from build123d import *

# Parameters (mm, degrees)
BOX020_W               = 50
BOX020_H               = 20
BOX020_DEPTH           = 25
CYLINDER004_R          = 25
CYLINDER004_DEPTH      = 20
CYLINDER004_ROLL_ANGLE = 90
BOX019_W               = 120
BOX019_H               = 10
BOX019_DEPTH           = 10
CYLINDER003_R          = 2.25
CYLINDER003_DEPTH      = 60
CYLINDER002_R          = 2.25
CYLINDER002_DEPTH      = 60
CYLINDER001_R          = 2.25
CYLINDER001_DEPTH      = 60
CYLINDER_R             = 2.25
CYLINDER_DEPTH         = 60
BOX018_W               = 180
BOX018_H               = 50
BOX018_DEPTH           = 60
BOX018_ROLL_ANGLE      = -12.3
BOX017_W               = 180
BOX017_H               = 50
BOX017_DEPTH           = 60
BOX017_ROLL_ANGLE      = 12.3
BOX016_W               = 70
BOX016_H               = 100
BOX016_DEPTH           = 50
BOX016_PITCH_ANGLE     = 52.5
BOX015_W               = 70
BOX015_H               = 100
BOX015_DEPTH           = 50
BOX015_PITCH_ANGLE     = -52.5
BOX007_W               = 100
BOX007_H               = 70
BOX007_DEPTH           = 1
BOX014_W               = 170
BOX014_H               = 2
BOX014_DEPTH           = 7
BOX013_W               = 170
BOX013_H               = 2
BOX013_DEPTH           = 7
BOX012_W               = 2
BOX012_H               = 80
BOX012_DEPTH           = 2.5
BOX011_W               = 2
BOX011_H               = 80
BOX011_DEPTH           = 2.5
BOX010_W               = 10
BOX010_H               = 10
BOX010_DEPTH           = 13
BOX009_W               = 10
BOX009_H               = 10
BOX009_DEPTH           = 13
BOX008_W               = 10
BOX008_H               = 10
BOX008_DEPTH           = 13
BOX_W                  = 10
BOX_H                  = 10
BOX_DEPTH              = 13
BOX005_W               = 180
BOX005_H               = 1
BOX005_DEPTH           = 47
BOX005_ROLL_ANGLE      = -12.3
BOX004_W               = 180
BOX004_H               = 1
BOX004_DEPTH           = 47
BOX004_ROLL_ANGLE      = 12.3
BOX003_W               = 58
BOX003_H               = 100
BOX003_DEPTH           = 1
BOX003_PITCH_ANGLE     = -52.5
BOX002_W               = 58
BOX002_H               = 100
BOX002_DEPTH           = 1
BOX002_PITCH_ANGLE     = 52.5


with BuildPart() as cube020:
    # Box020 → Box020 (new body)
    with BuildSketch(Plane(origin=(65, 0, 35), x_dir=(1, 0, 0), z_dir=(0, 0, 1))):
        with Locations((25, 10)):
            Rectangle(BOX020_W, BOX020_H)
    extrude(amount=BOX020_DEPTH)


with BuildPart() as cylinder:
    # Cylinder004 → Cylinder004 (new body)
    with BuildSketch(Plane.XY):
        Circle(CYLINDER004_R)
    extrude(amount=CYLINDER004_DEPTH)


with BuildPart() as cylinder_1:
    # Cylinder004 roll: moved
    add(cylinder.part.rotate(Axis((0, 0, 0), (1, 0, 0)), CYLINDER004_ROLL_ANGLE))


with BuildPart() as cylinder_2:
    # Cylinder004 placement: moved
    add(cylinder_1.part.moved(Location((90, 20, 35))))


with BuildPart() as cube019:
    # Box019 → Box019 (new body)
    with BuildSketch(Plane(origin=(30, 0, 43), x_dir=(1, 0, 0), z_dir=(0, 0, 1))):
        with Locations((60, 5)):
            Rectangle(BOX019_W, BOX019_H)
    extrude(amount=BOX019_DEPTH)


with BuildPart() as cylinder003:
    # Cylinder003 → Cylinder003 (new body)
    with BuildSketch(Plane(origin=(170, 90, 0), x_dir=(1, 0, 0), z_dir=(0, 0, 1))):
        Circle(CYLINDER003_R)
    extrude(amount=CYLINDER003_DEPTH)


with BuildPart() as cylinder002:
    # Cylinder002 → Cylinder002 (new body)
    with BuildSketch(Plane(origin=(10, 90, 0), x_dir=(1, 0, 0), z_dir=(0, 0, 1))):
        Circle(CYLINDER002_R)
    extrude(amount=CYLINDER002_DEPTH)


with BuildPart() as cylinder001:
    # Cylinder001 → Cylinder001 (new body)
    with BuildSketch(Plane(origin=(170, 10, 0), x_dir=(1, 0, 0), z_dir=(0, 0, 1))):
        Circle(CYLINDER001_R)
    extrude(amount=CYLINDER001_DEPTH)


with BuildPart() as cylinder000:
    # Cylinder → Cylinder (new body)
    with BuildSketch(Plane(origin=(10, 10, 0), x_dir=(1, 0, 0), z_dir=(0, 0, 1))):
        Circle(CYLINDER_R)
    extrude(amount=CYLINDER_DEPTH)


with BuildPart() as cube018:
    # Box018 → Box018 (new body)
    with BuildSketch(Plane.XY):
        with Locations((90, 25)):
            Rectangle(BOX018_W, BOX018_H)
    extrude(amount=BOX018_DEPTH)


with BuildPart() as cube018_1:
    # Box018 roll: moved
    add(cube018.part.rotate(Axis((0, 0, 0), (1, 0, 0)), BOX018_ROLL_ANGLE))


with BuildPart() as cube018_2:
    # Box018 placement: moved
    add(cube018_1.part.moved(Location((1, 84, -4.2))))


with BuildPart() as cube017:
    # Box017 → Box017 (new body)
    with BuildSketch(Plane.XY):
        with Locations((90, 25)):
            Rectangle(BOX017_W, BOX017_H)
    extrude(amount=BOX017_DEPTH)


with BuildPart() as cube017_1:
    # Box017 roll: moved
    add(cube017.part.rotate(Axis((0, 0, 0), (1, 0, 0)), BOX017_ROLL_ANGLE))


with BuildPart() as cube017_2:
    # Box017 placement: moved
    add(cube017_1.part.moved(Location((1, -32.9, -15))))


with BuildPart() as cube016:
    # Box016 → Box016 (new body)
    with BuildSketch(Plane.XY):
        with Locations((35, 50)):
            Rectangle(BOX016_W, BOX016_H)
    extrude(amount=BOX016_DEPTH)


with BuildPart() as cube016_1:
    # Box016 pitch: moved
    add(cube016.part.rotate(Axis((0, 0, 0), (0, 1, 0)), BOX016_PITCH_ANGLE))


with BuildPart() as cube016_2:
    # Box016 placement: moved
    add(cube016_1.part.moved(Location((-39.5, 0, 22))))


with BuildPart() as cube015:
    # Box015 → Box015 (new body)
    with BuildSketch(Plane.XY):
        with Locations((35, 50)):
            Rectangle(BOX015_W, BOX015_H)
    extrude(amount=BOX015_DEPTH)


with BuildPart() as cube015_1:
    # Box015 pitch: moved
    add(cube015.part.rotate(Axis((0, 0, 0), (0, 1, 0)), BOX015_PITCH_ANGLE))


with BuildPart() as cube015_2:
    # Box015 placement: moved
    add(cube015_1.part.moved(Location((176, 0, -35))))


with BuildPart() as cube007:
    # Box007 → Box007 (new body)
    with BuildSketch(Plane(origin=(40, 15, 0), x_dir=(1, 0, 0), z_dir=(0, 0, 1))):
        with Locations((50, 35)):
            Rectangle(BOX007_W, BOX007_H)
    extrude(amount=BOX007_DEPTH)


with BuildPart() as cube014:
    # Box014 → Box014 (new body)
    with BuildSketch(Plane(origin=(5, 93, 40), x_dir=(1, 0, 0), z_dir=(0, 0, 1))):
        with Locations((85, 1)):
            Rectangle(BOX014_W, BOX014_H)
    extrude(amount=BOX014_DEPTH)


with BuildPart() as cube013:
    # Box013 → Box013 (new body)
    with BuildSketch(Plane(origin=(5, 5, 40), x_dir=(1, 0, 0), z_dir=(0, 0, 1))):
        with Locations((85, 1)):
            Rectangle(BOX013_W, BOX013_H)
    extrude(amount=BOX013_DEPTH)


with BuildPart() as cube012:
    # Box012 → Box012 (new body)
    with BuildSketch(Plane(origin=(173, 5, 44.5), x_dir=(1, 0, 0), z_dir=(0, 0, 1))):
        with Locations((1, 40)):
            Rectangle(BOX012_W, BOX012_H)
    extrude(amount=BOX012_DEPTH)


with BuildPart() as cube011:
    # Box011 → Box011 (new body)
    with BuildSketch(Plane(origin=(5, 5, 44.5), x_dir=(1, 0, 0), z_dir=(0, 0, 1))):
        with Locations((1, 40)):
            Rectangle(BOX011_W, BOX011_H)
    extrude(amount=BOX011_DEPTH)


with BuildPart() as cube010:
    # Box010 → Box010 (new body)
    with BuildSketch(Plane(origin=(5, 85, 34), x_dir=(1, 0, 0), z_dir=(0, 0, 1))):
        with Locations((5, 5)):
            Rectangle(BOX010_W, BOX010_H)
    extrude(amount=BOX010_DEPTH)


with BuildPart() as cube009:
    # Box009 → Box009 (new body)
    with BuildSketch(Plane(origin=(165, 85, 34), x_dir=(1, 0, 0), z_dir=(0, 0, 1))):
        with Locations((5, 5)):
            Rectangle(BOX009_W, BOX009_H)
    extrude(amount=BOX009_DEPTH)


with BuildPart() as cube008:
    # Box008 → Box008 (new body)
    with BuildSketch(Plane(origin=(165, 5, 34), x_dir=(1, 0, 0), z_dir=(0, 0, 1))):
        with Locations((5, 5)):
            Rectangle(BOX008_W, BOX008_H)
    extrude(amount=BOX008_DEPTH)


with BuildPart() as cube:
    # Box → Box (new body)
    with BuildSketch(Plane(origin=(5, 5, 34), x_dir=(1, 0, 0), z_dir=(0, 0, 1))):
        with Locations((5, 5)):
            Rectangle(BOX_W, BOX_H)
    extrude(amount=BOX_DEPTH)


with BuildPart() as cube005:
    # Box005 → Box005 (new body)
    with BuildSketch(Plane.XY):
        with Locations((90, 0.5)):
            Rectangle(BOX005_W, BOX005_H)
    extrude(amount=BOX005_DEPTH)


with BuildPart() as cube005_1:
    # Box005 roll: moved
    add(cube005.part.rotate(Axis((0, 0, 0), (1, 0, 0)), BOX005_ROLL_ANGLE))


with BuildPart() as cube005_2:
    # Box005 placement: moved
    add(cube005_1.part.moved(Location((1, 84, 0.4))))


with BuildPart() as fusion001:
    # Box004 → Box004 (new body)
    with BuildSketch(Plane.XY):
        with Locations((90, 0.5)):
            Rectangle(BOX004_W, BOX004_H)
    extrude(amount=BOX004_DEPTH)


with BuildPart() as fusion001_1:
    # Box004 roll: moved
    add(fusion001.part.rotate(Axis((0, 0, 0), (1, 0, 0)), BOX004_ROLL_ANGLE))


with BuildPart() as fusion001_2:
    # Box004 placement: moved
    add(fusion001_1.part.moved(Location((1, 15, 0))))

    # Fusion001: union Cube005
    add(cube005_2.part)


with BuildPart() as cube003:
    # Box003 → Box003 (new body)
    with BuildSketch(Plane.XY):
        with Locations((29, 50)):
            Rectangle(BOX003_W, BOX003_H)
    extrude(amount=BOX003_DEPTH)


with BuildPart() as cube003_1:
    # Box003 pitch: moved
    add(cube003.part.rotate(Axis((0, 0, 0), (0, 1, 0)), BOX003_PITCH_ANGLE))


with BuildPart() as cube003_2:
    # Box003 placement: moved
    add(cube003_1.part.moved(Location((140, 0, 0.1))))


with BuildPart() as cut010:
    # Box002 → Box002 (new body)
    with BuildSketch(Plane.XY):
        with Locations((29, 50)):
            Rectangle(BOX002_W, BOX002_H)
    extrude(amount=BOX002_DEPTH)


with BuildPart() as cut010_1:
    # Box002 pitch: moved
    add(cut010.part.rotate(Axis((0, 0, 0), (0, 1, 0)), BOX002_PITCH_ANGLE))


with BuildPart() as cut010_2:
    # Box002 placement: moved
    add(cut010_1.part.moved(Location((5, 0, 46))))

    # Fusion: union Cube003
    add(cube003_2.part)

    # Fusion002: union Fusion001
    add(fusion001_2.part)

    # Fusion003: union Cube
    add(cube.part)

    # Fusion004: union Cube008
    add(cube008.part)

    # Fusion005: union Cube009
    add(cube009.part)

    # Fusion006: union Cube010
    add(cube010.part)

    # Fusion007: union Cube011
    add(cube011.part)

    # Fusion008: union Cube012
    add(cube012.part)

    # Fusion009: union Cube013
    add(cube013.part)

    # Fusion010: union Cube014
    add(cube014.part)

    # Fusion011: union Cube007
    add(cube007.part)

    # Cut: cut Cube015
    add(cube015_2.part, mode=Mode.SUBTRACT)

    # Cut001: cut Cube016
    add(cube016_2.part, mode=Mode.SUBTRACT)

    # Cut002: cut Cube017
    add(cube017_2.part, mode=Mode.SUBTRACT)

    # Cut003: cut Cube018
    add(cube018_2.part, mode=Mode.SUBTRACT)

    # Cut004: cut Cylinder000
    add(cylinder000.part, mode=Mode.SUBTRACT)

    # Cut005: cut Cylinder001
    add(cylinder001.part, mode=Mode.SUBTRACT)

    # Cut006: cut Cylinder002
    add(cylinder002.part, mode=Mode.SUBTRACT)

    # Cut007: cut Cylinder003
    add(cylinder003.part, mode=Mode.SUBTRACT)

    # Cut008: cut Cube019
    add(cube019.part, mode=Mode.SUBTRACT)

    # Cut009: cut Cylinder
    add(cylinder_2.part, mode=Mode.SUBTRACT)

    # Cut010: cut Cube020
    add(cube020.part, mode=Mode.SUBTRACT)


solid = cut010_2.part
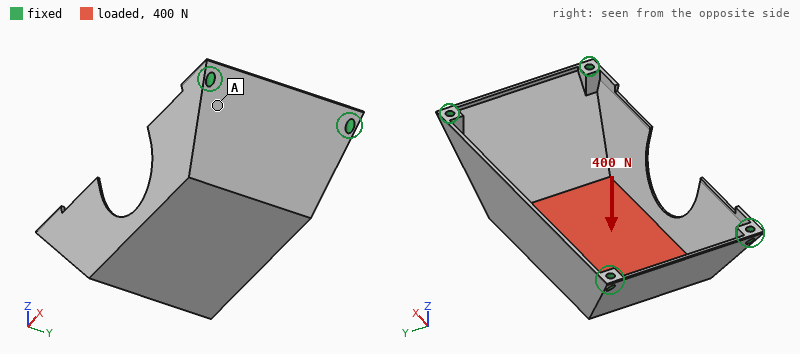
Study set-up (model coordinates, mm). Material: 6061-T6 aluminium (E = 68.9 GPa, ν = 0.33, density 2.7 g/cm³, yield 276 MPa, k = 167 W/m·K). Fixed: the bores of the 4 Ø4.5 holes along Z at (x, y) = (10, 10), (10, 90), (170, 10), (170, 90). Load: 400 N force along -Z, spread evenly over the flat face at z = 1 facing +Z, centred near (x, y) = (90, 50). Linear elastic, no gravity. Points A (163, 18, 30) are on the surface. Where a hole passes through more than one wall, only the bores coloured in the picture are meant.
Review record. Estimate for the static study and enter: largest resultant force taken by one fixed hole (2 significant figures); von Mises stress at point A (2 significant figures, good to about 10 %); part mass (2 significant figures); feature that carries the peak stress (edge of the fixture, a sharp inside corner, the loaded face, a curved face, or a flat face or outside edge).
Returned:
170 N
9.5 MPa
77 g
a flat face or outside edge
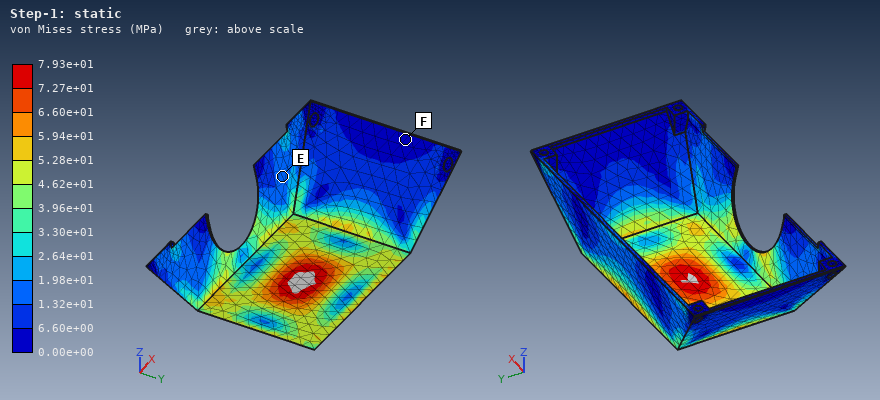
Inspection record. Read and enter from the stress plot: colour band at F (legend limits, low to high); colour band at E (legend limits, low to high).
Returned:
0.00e+00 to 6.60e+00 MPa
1.32e+01 to 1.98e+01 MPa
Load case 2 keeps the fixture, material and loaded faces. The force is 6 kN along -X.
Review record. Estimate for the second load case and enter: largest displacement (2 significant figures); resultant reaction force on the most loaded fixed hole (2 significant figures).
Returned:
0.14 mm
2.1 kN
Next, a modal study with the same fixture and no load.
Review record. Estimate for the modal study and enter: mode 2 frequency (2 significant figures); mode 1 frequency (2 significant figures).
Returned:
830 Hz
490 Hz
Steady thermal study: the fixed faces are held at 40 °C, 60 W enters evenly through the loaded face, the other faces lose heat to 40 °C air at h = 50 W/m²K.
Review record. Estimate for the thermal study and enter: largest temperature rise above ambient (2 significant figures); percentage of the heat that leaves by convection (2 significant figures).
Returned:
53 K
77 %
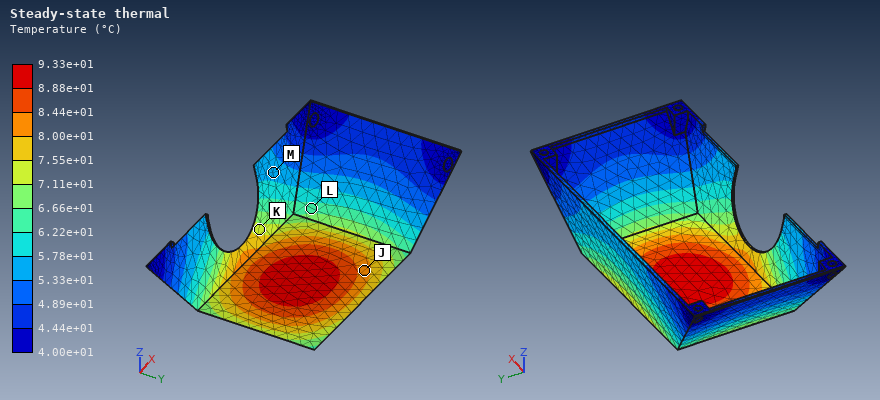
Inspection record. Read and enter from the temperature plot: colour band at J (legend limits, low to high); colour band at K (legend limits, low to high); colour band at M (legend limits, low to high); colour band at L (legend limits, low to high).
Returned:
8.00e+01 to 8.44e+01 °C
7.11e+01 to 7.55e+01 °C
5.33e+01 to 5.78e+01 °C
6.22e+01 to 6.66e+01 °C
